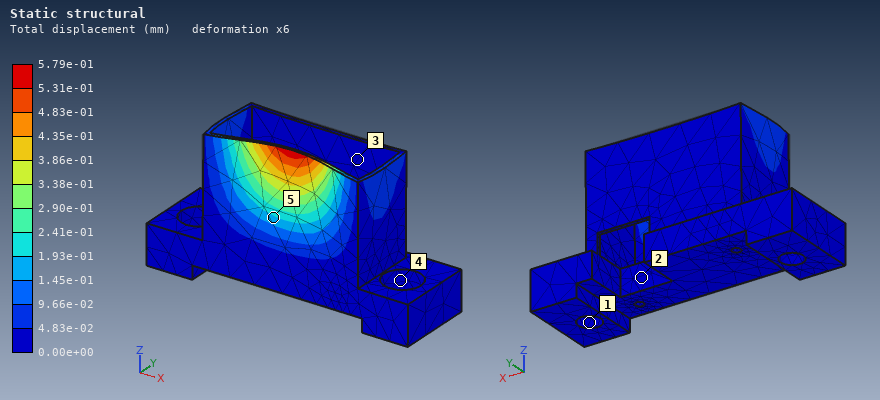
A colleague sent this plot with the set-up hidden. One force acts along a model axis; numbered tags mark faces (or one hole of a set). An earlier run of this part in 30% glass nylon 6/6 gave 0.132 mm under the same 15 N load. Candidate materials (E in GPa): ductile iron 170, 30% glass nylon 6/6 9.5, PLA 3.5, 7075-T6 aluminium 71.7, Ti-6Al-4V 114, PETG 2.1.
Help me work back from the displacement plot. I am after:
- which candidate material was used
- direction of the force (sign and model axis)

PETG
+Y
